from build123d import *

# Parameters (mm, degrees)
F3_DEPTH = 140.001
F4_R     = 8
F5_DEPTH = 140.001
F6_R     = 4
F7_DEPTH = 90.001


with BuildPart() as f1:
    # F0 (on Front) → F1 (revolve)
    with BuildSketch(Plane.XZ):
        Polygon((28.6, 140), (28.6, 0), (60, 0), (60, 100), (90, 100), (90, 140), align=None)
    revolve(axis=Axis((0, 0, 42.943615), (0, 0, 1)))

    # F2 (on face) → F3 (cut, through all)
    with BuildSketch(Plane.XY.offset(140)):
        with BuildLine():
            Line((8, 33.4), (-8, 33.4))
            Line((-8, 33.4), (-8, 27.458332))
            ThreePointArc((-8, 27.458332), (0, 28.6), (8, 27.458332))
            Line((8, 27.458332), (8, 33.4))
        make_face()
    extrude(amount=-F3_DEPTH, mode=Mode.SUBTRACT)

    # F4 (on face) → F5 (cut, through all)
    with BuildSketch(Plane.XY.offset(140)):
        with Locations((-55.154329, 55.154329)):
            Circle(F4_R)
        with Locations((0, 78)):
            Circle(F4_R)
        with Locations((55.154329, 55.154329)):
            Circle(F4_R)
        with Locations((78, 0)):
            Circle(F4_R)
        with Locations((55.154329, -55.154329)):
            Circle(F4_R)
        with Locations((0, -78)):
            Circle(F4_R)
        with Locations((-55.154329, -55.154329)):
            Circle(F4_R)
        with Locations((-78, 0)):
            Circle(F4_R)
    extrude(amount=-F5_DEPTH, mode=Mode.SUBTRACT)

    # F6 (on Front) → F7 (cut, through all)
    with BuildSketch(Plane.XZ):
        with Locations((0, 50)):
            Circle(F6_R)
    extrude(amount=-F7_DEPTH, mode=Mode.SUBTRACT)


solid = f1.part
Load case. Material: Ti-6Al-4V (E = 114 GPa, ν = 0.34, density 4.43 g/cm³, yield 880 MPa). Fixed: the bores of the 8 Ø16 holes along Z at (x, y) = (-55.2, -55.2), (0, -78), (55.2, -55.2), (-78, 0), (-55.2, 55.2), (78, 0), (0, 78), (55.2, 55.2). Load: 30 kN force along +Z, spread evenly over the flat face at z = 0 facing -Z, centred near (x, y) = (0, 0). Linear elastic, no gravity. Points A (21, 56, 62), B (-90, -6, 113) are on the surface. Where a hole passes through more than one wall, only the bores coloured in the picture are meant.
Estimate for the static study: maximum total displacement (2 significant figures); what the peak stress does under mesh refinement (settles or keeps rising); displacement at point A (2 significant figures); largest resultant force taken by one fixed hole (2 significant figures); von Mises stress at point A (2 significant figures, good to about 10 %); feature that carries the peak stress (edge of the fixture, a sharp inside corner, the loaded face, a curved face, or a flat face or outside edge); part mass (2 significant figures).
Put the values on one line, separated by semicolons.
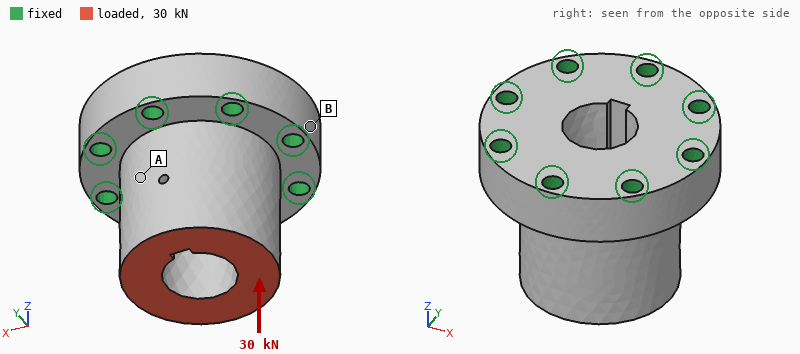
4.8 µm; keeps rising; 3.0 µm; 4.1 kN; 3.3 MPa; edge of the fixture; 7.6 kg
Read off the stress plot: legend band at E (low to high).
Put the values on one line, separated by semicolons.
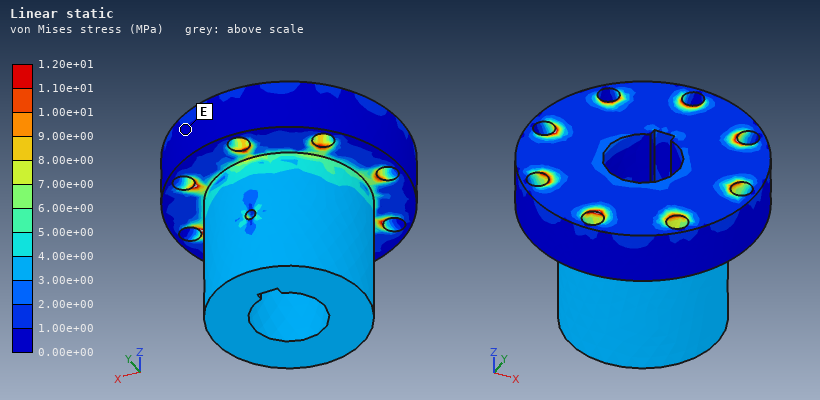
0.00e+00 to 1.00e+00 MPa
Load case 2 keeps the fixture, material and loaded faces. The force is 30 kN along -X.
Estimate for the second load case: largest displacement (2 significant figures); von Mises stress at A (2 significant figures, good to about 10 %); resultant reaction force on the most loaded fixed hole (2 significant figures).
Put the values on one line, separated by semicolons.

38 µm; 8.7 MPa; 14 kN
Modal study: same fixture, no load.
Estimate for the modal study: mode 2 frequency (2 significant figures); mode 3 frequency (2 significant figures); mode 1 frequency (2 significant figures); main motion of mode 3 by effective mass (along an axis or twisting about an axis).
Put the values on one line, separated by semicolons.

4100 Hz; 6700 Hz; 4100 Hz; twisting about Z
